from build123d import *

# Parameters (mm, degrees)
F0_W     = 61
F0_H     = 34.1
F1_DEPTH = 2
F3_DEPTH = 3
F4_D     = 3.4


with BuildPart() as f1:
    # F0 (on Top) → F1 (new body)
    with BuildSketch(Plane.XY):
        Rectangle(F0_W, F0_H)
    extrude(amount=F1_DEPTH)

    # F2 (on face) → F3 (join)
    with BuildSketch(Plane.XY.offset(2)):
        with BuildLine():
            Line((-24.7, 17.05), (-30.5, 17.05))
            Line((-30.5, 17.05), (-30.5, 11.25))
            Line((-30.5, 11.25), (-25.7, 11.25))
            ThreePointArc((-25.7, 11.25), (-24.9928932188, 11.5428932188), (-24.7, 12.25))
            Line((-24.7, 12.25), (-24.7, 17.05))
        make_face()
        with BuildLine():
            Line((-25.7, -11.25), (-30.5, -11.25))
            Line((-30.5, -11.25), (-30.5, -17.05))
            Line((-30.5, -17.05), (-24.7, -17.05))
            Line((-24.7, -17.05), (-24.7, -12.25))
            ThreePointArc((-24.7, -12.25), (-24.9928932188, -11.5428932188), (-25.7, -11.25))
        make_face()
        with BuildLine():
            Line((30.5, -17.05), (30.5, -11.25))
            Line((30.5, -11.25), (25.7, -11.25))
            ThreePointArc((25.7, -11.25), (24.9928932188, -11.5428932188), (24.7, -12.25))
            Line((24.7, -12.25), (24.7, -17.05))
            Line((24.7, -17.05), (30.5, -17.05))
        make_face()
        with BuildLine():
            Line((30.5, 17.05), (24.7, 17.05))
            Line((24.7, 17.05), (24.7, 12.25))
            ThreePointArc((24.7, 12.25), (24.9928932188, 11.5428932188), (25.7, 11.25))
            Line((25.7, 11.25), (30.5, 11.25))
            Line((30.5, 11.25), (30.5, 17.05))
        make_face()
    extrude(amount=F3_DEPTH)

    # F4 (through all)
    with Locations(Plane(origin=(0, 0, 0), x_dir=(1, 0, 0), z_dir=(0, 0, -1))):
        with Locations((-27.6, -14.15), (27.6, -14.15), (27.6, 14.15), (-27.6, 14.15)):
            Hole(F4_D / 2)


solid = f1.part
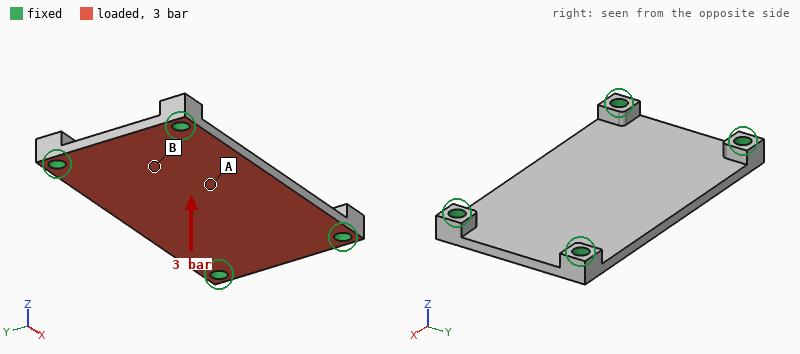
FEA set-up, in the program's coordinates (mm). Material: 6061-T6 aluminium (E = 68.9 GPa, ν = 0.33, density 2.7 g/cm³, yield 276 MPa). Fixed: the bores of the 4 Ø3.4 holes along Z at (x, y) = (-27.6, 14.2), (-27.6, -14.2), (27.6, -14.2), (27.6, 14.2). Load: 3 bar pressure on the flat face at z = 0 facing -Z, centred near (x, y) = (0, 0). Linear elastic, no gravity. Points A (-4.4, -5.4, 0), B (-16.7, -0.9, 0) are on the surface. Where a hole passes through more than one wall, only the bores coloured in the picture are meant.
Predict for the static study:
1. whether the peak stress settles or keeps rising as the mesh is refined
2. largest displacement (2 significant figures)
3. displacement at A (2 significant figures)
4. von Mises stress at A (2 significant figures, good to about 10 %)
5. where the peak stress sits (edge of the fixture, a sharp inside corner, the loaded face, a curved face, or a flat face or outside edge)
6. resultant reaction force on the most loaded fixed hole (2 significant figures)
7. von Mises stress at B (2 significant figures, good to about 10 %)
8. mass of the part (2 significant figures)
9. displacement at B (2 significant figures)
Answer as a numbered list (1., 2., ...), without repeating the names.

1. keeps rising
2. 0.16 mm
3. 0.15 mm
4. 47 MPa
5. a sharp inside corner
6. 160 N
7. 18 MPa
8. 12 g
9. 0.074 mm
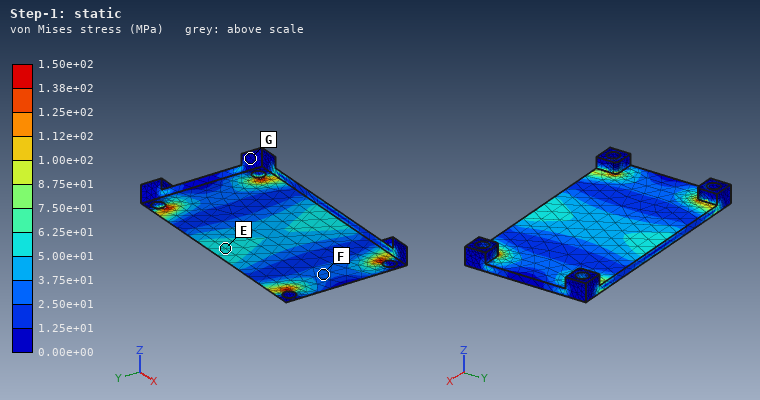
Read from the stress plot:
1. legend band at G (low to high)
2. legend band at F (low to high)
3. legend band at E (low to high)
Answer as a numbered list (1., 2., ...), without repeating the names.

1. 0.00e+00 to 1.25e+01 MPa
2. 2.50e+01 to 3.75e+01 MPa
3. 5.00e+01 to 6.25e+01 MPa
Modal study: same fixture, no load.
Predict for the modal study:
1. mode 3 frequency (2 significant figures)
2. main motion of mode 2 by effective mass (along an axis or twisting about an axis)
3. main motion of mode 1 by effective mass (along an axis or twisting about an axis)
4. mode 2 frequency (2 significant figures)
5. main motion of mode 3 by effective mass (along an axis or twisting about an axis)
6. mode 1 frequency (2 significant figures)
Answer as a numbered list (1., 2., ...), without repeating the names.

1. 9200 Hz
2. twisting about X
3. along Z
4. 5400 Hz
5. twisting about Y
6. 3400 Hz
